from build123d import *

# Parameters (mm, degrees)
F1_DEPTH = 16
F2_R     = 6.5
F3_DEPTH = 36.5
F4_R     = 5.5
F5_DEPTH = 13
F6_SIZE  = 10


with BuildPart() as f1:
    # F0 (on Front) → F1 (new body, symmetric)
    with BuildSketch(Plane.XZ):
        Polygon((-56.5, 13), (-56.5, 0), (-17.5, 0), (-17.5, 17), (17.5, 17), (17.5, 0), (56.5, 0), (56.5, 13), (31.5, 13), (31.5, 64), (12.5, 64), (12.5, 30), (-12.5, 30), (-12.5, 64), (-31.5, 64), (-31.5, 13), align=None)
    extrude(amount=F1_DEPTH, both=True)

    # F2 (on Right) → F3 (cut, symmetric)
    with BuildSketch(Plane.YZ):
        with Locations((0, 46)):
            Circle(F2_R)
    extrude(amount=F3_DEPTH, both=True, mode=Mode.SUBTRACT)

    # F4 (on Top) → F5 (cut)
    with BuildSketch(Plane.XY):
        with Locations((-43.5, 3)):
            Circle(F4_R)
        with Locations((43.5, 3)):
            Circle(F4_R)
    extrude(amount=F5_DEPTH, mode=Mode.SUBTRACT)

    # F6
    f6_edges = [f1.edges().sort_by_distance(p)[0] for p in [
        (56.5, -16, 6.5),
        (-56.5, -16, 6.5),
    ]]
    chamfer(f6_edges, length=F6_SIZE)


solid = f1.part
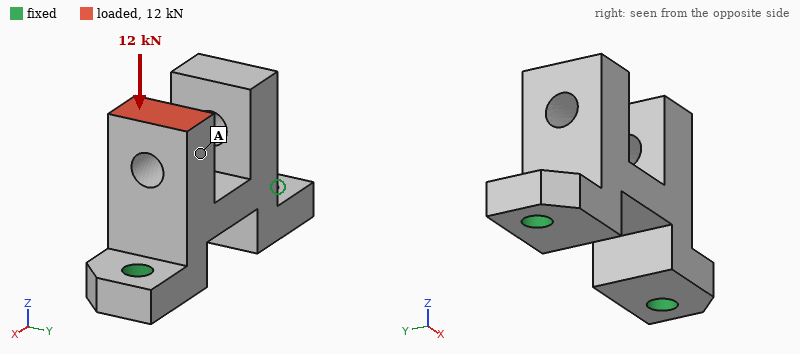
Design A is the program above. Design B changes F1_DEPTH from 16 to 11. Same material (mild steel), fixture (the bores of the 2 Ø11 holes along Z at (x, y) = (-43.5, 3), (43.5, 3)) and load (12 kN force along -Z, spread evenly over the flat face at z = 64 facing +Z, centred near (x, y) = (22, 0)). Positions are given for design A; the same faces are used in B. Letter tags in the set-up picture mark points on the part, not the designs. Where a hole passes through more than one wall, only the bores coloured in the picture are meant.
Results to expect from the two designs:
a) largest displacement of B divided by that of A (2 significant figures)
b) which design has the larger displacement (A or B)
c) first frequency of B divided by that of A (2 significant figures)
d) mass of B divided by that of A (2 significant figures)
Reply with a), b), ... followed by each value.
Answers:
a) 1.3
b) B
c) 0.94
d) 0.66
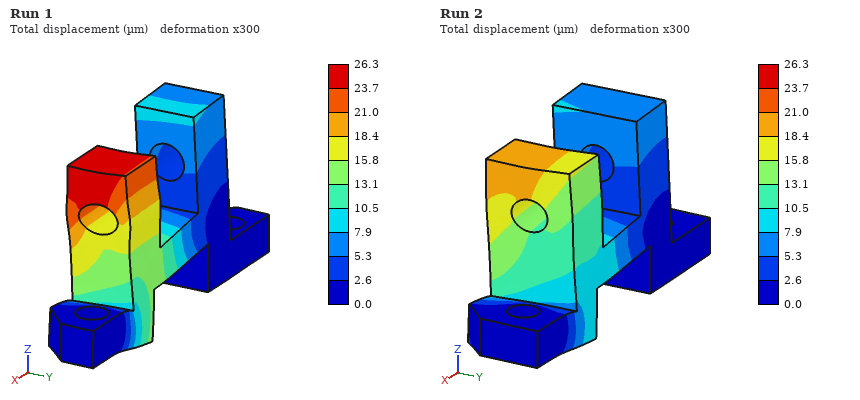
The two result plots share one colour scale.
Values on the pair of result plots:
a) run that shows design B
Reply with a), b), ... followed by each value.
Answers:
a) Run 1
